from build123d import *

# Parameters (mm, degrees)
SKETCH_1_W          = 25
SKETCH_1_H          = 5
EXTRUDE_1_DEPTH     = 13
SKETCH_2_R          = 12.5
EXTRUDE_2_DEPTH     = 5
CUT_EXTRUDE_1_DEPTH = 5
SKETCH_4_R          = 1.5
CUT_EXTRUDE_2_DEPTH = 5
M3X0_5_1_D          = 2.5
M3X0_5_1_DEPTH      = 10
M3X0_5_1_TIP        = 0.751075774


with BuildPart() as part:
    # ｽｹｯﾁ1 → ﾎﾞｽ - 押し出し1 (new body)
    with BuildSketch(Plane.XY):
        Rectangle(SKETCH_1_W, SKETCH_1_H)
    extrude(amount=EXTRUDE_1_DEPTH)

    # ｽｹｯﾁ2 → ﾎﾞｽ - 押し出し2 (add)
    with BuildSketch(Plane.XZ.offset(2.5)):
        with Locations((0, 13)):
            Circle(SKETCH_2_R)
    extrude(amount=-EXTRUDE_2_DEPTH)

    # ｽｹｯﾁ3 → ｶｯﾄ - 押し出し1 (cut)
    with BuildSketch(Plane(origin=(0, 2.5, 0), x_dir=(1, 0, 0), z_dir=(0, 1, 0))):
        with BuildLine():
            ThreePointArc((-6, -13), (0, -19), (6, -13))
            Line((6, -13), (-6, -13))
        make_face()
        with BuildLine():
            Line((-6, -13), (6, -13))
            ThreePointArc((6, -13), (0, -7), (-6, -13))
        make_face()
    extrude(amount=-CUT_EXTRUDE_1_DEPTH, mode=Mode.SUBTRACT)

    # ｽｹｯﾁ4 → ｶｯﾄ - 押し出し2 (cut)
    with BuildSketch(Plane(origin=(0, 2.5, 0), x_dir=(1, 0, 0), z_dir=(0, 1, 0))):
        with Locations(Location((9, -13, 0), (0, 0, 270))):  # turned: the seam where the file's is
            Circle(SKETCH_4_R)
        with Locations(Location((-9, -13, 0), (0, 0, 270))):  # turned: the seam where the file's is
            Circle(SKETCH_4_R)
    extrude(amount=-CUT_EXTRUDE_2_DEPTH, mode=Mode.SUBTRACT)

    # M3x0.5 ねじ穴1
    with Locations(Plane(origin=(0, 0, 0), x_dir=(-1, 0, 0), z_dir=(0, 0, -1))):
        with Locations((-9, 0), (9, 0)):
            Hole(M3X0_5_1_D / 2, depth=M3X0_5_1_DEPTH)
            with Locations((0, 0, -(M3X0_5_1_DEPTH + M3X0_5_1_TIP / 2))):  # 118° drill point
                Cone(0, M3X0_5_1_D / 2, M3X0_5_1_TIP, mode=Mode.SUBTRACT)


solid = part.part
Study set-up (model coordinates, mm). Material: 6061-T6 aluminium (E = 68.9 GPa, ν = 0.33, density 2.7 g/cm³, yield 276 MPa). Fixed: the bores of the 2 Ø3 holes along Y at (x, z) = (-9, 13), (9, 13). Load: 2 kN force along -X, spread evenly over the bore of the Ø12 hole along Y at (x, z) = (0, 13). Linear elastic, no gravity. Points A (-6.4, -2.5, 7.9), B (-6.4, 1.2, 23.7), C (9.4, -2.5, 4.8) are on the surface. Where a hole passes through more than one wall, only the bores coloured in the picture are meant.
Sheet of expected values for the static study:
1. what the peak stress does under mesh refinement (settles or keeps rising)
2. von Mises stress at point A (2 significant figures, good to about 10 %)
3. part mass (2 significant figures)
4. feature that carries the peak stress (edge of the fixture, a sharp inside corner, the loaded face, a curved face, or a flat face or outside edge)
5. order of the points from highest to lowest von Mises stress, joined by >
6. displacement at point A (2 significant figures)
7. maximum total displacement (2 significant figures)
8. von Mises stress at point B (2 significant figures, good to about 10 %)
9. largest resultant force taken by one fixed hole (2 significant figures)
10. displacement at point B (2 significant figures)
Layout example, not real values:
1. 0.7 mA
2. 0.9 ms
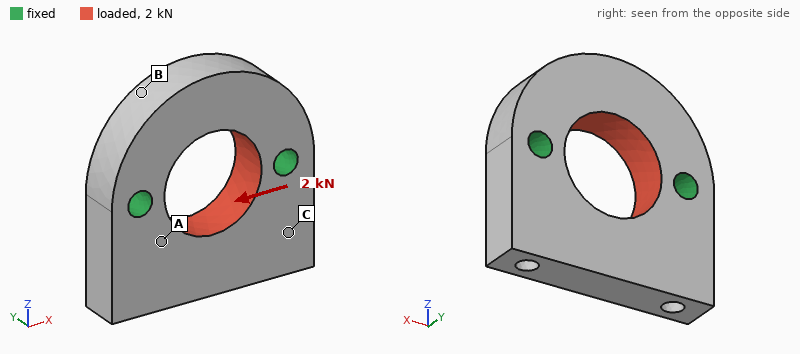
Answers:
1. keeps rising
2. 18 MPa
3. 5.7 g
4. edge of the fixture
5. A > B > C
6. 3.2 µm
7. 4.7 µm
8. 10 MPa
9. 1.0 kN
10. 3.8 µm
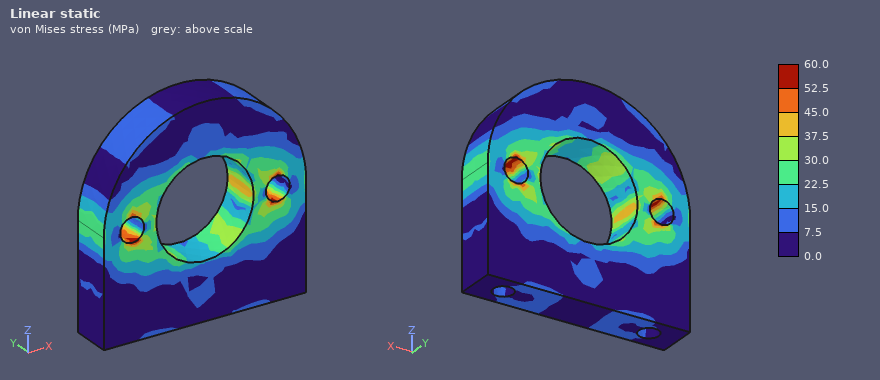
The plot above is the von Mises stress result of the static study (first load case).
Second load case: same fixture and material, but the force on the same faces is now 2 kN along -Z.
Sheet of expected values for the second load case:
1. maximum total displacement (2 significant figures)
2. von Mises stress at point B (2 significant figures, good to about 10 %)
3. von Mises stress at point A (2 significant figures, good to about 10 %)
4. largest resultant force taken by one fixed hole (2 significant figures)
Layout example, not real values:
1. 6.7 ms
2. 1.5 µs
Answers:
1. 3.7 µm
2. 9.7 MPa
3. 16 MPa
4. 1.0 kN
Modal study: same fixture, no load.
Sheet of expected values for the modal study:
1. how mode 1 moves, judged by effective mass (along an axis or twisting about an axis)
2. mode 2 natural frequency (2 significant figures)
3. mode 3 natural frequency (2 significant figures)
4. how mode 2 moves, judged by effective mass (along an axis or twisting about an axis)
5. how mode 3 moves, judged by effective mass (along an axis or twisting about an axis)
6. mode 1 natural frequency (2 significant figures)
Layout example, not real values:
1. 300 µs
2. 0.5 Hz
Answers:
1. along Y
2. 23 kHz
3. 31 kHz
4. along Y
5. twisting about Z
6. 18 kHz
